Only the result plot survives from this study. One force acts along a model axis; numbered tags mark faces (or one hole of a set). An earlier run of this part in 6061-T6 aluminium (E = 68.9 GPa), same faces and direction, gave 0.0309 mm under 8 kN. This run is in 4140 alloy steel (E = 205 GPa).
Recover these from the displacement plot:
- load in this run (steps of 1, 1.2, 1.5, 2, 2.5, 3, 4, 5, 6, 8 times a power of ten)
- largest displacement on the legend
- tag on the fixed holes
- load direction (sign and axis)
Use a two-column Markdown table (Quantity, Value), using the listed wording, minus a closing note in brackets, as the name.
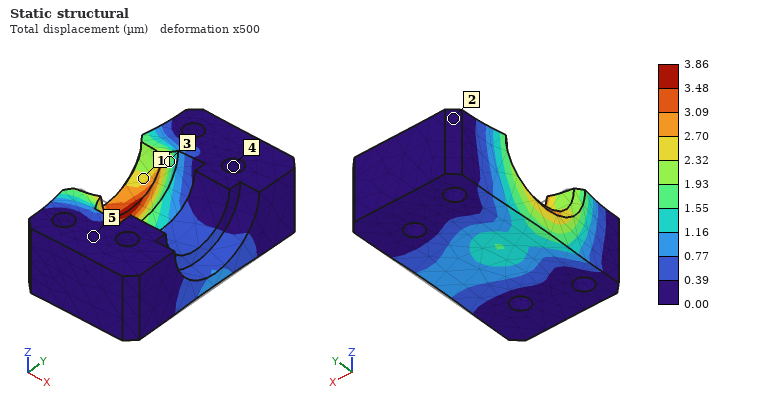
| Quantity | Value |
|---|---|
| load in this run | 3 kN |
| largest displacement on the legend | 3.86 µm |
| tag on the fixed holes | 4 |
| load direction | -X |
